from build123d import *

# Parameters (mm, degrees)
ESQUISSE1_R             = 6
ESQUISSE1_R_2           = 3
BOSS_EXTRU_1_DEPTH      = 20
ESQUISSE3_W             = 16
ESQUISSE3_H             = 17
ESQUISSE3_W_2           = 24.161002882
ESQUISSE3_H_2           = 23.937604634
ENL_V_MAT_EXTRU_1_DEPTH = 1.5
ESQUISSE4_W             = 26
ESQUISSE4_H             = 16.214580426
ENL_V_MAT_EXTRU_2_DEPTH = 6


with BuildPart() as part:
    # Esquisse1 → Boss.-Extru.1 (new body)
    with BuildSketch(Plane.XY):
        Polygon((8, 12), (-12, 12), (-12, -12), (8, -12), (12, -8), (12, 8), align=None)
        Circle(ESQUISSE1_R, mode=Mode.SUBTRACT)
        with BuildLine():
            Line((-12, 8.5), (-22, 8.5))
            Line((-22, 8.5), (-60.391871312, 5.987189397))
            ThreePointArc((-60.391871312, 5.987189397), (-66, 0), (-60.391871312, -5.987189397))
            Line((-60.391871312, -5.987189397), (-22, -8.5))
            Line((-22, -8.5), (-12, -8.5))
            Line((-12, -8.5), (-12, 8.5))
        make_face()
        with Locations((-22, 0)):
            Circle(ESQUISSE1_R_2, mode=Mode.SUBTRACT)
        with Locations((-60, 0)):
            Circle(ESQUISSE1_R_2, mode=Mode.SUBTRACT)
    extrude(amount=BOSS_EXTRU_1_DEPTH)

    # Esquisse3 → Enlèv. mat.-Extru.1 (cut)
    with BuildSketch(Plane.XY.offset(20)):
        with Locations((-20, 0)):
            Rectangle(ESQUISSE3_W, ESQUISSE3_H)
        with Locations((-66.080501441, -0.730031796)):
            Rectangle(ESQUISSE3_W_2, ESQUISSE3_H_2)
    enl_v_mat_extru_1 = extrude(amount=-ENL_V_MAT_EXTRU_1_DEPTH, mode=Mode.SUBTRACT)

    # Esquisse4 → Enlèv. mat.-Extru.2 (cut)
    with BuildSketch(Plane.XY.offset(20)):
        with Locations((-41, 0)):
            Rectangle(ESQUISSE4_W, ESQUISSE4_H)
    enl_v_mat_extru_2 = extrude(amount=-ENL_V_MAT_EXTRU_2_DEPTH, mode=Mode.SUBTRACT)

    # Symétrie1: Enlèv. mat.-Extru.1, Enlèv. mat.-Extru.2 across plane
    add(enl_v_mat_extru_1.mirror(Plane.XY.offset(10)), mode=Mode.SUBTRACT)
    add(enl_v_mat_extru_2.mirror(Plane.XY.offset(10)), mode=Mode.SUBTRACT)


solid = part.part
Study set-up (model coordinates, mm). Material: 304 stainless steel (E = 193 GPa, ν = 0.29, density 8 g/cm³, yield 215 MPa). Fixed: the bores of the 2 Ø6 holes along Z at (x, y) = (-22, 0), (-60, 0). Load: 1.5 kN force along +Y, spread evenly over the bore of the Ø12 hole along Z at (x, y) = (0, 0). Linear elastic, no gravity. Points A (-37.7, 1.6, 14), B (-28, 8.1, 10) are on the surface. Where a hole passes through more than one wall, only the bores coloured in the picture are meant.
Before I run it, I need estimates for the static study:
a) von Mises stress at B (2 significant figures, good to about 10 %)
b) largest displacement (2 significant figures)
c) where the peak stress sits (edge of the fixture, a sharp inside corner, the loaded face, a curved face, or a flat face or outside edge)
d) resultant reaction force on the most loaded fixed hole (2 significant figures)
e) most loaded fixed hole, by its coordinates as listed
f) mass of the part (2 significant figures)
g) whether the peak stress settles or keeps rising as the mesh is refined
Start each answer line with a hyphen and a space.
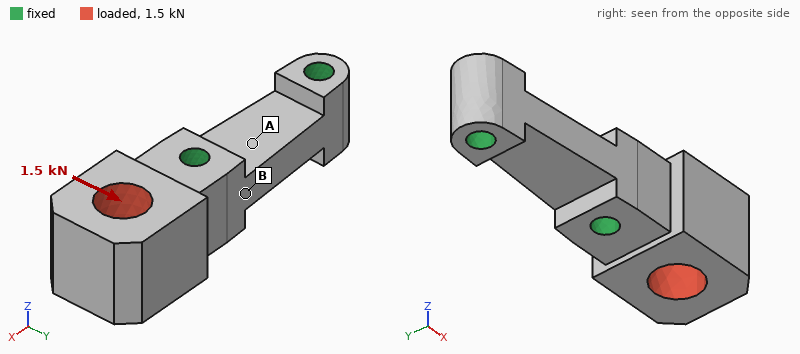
- 13 MPa
- 14 µm
- edge of the fixture
- 1.7 kN
- (-22, 0)
- 140 g
- keeps rising
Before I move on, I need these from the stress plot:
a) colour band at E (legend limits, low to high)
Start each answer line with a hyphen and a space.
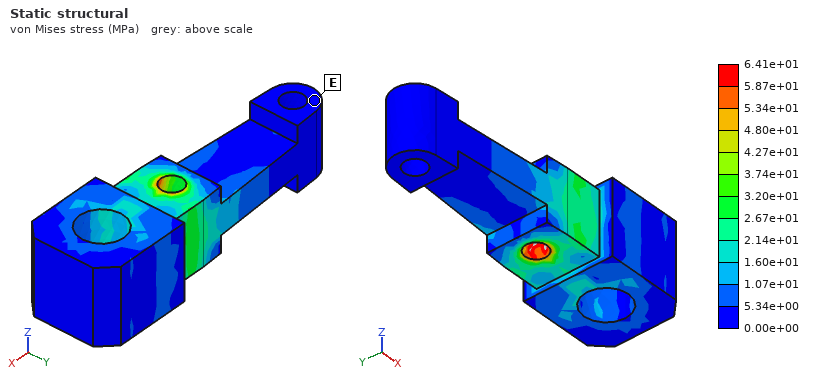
- 0.00e+00 to 5.34e+00 MPa
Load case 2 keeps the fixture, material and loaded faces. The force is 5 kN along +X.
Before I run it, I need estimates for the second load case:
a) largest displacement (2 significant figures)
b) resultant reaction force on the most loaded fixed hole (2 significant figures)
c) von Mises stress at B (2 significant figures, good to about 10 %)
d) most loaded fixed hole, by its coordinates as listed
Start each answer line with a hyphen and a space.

- 3.6 µm
- 4.9 kN
- 5.0 MPa
- (-22, 0)
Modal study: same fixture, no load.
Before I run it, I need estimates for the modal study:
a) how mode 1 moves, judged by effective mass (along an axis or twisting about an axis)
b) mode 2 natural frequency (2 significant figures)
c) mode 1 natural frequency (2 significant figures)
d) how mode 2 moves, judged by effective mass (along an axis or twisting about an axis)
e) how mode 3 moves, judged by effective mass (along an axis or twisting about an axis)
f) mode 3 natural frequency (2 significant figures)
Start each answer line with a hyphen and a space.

- along Y
- 9000 Hz
- 7000 Hz
- along Z
- twisting about X
- 16 kHz
